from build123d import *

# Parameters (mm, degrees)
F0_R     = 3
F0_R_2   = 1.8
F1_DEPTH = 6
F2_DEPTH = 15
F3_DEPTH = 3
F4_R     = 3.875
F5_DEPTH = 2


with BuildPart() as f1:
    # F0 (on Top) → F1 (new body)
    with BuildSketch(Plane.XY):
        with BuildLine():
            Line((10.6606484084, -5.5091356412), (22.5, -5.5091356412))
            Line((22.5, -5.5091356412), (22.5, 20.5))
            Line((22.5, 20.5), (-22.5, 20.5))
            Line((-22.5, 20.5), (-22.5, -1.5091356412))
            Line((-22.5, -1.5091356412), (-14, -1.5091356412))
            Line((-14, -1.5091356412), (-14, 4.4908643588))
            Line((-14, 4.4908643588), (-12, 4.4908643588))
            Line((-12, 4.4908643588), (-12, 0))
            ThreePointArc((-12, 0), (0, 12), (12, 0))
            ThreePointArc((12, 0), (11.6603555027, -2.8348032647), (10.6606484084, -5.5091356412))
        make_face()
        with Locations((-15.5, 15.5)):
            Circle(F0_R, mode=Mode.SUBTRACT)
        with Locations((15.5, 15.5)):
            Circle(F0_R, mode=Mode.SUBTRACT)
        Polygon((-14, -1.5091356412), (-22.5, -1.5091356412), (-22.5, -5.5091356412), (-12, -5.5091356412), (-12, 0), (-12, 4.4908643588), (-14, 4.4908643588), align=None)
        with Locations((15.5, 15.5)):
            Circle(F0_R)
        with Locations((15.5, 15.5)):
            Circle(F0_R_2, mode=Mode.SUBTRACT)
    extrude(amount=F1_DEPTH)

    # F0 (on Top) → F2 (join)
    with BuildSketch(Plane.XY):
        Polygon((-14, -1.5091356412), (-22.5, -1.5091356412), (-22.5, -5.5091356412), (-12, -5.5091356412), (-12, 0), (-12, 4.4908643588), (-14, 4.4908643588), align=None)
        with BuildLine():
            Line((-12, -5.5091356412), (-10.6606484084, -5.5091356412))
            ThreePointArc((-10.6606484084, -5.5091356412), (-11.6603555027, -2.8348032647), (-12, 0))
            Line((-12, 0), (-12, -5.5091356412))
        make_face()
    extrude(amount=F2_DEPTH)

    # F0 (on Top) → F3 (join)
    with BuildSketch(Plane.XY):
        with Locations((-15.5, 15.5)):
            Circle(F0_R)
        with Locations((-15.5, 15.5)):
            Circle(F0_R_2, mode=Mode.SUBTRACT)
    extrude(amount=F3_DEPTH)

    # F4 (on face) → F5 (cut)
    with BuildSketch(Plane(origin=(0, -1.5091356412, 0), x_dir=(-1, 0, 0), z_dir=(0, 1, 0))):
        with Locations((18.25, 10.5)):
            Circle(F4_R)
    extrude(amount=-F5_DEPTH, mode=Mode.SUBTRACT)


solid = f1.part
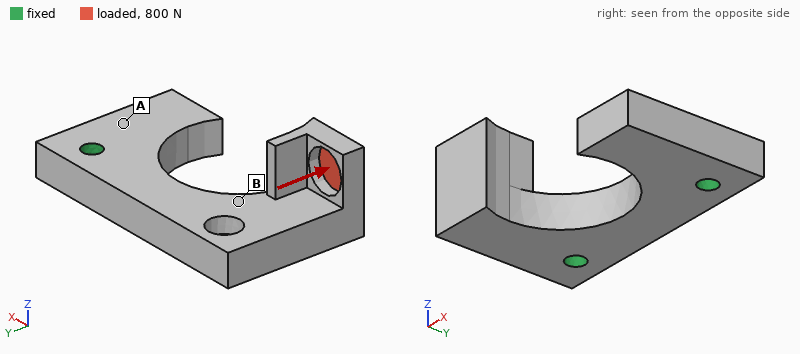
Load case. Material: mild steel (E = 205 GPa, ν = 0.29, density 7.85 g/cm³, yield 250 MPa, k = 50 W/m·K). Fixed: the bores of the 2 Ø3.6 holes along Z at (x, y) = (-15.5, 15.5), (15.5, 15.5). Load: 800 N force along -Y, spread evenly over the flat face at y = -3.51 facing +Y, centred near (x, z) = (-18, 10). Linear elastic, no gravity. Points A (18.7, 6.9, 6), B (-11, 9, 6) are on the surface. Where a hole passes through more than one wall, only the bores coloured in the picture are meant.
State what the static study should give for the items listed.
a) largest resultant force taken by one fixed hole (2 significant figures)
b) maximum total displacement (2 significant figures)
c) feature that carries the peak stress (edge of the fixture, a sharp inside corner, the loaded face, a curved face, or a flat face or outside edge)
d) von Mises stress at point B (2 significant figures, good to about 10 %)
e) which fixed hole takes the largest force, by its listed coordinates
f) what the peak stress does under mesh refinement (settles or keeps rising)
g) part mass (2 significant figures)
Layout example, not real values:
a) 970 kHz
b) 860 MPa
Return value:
a) 810 N
b) 75 µm
c) edge of the fixture
d) 88 MPa
e) (-15.5, 15.5)
f) keeps rising
g) 40 g
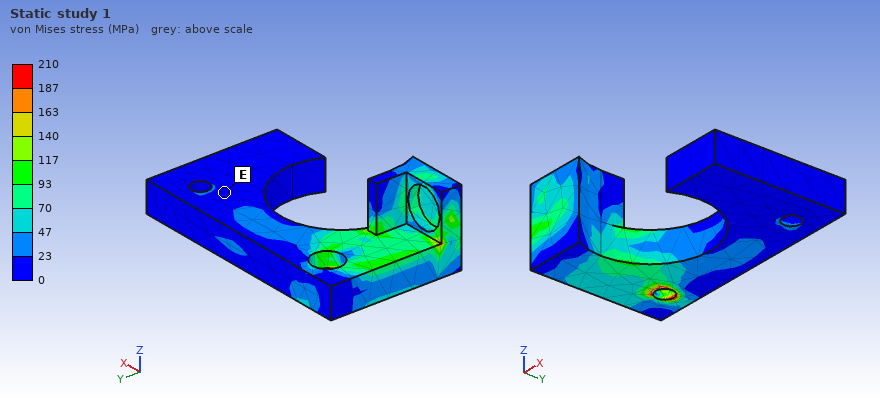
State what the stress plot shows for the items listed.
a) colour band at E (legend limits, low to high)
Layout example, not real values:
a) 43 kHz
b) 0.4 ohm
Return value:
a) 0 to 23 MPa
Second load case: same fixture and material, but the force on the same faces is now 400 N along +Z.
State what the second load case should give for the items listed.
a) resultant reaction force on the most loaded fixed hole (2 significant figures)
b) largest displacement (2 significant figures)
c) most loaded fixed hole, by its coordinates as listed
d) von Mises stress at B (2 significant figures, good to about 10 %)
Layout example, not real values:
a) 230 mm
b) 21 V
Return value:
a) 440 N
b) 52 µm
c) (-15.5, 15.5)
d) 78 MPa
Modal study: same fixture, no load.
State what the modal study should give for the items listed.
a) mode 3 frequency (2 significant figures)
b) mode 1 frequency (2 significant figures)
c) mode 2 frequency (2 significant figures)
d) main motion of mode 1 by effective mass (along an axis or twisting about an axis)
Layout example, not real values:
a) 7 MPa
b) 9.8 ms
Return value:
a) 12 kHz
b) 5900 Hz
c) 10 kHz
d) along Z
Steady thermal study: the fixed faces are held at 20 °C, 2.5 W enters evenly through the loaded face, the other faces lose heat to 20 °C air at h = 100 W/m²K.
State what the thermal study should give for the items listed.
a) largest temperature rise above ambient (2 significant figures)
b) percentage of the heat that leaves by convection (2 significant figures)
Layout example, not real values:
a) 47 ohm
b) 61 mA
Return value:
a) 17 K
b) 39 %
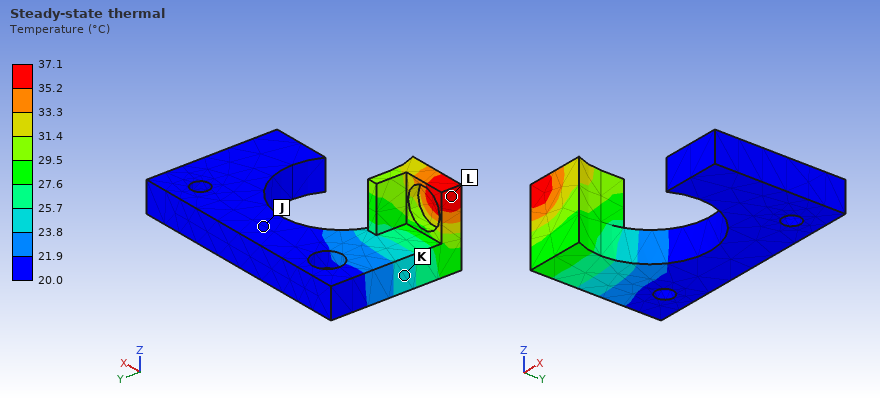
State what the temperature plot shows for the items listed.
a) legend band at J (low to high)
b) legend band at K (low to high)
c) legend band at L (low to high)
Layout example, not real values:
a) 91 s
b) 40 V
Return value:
a) 20.0 to 21.9 °C
b) 23.8 to 25.7 °C
c) 35.2 to 37.1 °C
